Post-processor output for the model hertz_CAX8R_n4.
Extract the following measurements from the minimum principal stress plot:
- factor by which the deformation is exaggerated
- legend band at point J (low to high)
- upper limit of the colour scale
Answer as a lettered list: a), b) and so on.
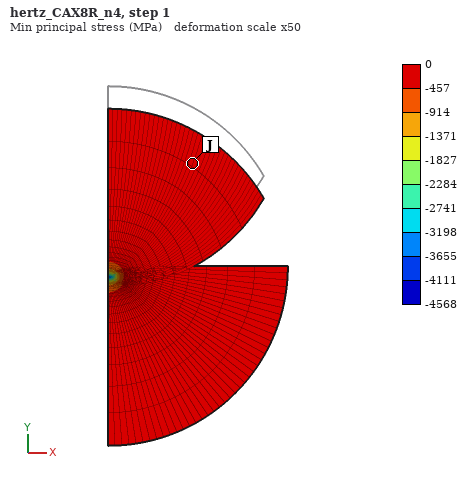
a) 50
b) -457 to 0 MPa
c) 0 MPa
